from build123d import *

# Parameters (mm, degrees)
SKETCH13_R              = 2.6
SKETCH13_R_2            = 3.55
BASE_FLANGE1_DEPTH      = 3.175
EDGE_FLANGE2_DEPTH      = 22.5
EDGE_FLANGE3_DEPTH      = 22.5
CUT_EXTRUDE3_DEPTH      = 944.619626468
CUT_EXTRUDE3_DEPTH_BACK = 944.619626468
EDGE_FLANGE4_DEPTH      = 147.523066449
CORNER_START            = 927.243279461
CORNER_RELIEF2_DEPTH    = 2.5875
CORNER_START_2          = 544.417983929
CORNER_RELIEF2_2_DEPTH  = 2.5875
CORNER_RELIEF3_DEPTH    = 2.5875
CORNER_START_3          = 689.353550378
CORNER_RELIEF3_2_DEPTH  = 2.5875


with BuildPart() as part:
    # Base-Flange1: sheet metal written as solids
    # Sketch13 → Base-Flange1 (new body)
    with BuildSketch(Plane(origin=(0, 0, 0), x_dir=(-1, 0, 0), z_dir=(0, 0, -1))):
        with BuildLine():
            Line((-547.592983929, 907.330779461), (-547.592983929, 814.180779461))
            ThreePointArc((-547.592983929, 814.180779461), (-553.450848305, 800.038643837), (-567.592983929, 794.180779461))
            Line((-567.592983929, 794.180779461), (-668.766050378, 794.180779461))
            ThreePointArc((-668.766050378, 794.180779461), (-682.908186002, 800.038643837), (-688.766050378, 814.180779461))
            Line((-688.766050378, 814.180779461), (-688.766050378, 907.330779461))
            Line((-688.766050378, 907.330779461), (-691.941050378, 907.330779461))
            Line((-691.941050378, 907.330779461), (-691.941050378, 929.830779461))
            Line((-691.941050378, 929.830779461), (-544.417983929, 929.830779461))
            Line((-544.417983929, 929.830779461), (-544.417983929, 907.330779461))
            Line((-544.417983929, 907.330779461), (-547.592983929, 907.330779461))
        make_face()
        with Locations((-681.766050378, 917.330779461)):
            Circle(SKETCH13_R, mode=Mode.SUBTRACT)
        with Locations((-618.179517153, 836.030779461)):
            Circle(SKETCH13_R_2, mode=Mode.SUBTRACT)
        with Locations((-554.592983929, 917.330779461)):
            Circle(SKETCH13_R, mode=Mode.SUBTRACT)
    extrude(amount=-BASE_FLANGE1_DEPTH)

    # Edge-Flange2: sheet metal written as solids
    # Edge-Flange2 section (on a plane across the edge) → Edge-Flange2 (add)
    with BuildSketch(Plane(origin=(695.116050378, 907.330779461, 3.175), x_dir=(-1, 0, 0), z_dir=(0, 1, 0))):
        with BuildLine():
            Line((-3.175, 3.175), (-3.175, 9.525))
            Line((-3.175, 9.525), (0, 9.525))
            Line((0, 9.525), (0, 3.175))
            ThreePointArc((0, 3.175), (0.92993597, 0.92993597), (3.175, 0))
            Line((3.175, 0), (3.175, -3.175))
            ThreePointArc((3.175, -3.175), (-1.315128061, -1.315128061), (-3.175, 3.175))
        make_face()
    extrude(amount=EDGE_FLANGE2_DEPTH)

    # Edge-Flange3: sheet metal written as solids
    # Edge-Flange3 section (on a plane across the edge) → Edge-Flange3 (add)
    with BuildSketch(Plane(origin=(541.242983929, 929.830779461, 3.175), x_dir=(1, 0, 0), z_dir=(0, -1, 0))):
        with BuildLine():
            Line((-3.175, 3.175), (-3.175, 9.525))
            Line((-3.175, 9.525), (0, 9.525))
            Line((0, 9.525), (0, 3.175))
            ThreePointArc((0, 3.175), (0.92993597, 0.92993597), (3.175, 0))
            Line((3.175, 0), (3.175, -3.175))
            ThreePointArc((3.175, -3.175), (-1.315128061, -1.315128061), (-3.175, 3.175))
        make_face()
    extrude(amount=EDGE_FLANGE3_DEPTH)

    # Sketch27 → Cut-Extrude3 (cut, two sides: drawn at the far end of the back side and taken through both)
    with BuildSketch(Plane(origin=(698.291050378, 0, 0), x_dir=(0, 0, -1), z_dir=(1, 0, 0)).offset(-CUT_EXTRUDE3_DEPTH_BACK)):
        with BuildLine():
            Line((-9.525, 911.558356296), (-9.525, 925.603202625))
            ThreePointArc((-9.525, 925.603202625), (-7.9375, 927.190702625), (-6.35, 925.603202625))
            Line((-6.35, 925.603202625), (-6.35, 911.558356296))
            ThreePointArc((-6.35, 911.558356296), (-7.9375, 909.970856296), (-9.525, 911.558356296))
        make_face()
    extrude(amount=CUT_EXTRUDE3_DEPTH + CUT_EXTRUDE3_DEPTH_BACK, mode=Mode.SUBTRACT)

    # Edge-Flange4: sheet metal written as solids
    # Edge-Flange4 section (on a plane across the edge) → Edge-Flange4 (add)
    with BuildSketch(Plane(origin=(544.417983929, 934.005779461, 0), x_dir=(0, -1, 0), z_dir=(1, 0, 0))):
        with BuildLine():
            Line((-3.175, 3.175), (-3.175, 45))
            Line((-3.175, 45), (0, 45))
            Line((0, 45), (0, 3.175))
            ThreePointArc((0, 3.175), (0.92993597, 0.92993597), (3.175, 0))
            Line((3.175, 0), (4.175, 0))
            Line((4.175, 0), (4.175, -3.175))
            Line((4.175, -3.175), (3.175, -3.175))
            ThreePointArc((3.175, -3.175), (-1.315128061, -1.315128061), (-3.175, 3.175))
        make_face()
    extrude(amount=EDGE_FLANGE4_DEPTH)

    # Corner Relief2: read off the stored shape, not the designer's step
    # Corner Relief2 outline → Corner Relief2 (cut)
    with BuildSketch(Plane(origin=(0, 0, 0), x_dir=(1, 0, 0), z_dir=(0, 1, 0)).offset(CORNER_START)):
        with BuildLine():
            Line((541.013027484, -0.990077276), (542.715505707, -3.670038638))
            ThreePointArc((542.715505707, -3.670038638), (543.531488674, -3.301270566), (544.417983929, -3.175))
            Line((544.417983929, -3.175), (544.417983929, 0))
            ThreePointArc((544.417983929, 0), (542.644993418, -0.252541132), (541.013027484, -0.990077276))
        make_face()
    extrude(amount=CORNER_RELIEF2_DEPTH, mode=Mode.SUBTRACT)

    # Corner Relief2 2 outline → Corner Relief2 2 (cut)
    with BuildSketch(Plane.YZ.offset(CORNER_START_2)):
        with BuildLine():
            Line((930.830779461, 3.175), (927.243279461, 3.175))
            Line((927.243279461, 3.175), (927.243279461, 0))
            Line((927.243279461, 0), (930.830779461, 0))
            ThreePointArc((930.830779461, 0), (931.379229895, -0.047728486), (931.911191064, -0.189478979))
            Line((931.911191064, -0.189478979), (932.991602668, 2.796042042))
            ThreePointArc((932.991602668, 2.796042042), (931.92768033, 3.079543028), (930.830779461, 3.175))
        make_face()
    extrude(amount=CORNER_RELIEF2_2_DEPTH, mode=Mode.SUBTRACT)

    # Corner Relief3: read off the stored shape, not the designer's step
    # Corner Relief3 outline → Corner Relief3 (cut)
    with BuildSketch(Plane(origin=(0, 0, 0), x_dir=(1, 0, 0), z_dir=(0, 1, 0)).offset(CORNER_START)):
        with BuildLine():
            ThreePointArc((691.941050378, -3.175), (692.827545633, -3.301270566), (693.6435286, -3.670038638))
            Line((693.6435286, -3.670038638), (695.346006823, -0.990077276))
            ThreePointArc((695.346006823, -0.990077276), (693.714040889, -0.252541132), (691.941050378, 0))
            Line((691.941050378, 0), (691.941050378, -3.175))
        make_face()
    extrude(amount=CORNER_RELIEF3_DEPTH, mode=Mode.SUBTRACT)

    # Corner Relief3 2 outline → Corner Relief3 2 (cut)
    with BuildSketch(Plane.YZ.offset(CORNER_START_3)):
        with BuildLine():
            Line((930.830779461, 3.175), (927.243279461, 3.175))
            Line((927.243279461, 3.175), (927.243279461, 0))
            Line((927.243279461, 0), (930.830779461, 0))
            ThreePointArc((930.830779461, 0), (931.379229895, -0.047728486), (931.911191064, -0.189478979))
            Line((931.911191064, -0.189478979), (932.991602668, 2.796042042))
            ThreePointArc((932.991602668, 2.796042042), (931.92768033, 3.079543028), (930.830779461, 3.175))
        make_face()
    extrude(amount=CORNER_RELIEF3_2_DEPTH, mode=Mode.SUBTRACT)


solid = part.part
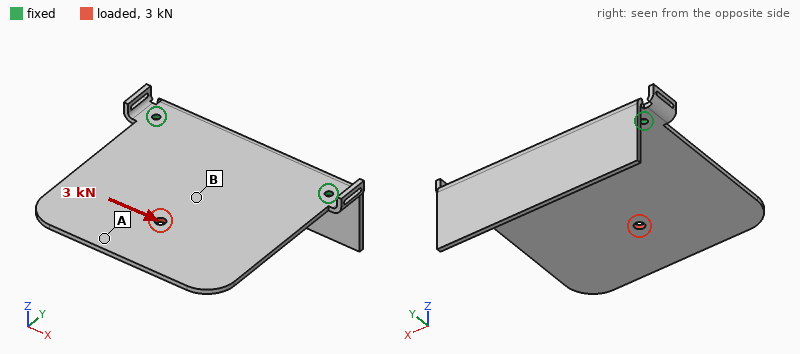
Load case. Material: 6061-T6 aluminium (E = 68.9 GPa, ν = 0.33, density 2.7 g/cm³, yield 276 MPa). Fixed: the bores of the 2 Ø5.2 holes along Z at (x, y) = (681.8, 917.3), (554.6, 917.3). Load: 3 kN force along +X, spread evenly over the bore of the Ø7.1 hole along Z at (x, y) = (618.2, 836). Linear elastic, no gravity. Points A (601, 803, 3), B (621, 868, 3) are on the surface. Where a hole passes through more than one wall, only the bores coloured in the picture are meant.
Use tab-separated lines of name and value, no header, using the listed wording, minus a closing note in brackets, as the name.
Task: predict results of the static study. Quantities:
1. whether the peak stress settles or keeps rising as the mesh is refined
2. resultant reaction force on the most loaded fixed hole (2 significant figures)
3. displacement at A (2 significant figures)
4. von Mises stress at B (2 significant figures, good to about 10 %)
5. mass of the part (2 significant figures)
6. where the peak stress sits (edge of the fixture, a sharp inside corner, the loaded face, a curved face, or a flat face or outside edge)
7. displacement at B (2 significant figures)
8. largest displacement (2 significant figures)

whether the peak stress settles or keeps rising as the mesh is refined	keeps rising
resultant reaction force on the most loaded fixed hole	2.4 kN
displacement at A	48 µm
von Mises stress at B	14 MPa
mass of the part	230 g
where the peak stress sits	edge of the fixture
displacement at B	24 µm
largest displacement	52 µm
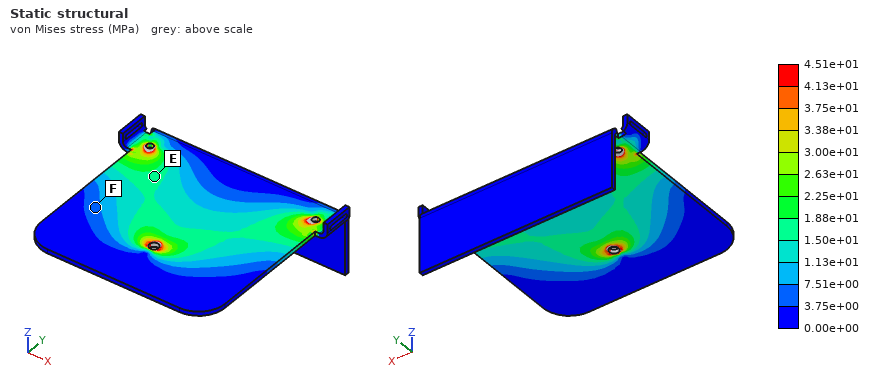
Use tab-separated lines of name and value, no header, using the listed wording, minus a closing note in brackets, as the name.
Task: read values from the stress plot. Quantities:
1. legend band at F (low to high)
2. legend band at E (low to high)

legend band at F	3.75e+00 to 7.51e+00 MPa
legend band at E	1.50e+01 to 1.88e+01 MPa
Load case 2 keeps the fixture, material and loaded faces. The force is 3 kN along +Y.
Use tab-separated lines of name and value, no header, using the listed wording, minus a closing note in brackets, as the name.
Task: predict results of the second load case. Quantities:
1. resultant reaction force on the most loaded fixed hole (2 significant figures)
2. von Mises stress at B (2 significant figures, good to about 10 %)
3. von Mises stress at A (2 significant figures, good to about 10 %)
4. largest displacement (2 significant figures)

resultant reaction force on the most loaded fixed hole	1.6 kN
von Mises stress at B	9.8 MPa
von Mises stress at A	6.9 MPa
largest displacement	27 µm
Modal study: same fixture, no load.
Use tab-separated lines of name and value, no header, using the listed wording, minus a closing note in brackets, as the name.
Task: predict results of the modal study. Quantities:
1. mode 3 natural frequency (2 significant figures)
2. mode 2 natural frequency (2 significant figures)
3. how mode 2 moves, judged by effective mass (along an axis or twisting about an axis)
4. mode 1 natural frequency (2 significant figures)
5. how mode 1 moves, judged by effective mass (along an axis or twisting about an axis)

mode 3 natural frequency	660 Hz
mode 2 natural frequency	400 Hz
how mode 2 moves, judged by effective mass	twisting about Y
mode 1 natural frequency	140 Hz
how mode 1 moves, judged by effective mass	along Z
